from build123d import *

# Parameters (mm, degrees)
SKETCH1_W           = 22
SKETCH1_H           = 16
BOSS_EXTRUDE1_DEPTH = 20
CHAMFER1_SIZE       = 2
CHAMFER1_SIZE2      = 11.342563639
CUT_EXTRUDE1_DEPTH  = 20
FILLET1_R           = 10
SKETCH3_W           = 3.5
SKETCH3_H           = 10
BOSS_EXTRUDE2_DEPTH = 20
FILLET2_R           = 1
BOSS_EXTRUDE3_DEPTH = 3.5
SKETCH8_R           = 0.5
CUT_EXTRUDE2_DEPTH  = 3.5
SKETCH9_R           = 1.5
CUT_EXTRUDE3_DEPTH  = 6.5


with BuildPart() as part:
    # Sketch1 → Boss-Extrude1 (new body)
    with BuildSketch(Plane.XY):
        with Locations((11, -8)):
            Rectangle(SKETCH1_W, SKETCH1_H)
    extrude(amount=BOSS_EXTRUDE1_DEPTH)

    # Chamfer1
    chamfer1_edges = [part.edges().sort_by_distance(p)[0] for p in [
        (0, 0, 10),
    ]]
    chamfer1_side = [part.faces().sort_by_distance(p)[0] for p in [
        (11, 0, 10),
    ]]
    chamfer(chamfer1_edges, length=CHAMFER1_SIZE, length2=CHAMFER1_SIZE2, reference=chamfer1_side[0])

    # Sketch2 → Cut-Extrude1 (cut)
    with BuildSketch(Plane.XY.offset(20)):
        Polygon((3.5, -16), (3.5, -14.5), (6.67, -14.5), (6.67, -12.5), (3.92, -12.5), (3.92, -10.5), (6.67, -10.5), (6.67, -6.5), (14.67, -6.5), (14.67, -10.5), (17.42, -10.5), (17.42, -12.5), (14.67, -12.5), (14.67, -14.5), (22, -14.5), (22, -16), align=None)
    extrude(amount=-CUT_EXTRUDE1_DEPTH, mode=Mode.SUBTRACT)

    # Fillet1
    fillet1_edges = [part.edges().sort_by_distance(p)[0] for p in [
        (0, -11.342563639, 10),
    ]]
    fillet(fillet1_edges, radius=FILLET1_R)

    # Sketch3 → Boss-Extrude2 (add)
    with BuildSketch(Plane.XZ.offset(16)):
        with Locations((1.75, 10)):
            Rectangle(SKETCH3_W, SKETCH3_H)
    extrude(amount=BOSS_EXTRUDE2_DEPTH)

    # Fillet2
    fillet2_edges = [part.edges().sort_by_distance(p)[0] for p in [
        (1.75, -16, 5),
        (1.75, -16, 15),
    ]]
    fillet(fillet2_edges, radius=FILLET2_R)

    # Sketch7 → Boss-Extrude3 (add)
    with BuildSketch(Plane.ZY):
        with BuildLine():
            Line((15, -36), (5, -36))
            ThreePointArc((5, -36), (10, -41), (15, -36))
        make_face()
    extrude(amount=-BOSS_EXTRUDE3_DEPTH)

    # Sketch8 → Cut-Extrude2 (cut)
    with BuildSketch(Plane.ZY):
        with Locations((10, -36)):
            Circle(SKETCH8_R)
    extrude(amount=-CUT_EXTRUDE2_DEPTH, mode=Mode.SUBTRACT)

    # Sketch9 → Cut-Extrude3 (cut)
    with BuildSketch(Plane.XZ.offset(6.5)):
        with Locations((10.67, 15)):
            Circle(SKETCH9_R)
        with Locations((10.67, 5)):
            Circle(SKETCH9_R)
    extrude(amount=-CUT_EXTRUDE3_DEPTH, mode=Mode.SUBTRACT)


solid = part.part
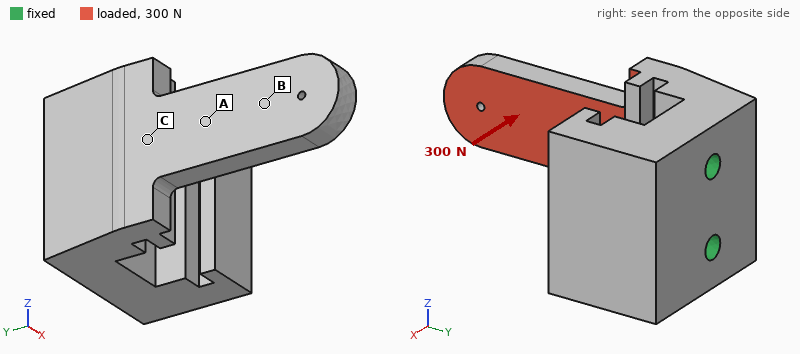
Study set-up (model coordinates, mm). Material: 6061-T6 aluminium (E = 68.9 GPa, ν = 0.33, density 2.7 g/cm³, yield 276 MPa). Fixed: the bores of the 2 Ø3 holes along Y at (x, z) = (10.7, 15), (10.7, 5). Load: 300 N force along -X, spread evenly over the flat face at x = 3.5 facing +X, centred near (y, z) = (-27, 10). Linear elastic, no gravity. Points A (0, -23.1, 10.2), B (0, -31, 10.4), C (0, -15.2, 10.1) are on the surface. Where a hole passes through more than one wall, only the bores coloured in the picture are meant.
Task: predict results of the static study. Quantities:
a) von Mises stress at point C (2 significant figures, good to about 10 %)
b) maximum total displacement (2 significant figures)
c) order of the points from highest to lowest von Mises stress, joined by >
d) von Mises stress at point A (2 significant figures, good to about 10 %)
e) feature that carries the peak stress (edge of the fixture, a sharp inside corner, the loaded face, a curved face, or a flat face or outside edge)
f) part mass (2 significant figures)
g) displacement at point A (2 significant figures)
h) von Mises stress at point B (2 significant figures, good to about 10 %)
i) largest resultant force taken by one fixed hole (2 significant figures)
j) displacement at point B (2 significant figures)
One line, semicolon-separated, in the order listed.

130 MPa; 0.46 mm; C > A > B; 76 MPa; a curved face; 15 g; 0.15 mm; 23 MPa; 180 N; 0.28 mm
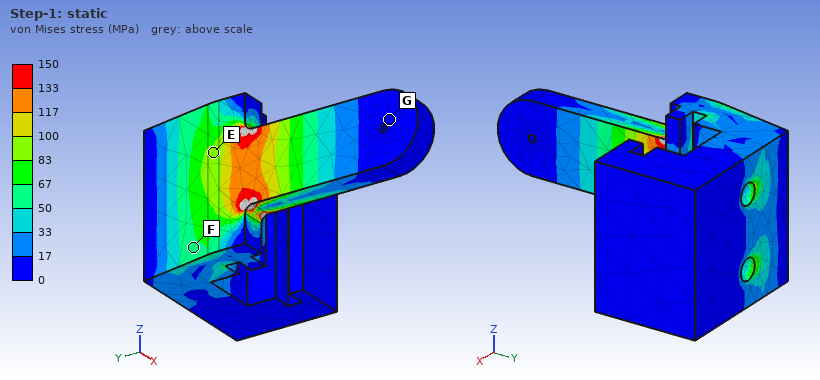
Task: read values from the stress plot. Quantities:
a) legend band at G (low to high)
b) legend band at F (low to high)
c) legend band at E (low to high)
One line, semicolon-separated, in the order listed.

0 to 17 MPa; 50 to 67 MPa; 83 to 100 MPa
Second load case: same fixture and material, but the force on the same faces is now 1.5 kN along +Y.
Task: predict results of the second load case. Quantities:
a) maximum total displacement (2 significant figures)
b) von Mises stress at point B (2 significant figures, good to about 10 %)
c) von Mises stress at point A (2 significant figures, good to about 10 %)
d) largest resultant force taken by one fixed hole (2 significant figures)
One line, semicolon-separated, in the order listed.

0.23 mm; 28 MPa; 52 MPa; 750 N
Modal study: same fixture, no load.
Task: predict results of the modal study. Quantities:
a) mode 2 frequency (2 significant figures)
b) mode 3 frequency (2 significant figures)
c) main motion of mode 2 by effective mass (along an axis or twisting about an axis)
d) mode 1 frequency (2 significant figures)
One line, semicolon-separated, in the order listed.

8000 Hz; 14 kHz; along Z; 3200 Hz
